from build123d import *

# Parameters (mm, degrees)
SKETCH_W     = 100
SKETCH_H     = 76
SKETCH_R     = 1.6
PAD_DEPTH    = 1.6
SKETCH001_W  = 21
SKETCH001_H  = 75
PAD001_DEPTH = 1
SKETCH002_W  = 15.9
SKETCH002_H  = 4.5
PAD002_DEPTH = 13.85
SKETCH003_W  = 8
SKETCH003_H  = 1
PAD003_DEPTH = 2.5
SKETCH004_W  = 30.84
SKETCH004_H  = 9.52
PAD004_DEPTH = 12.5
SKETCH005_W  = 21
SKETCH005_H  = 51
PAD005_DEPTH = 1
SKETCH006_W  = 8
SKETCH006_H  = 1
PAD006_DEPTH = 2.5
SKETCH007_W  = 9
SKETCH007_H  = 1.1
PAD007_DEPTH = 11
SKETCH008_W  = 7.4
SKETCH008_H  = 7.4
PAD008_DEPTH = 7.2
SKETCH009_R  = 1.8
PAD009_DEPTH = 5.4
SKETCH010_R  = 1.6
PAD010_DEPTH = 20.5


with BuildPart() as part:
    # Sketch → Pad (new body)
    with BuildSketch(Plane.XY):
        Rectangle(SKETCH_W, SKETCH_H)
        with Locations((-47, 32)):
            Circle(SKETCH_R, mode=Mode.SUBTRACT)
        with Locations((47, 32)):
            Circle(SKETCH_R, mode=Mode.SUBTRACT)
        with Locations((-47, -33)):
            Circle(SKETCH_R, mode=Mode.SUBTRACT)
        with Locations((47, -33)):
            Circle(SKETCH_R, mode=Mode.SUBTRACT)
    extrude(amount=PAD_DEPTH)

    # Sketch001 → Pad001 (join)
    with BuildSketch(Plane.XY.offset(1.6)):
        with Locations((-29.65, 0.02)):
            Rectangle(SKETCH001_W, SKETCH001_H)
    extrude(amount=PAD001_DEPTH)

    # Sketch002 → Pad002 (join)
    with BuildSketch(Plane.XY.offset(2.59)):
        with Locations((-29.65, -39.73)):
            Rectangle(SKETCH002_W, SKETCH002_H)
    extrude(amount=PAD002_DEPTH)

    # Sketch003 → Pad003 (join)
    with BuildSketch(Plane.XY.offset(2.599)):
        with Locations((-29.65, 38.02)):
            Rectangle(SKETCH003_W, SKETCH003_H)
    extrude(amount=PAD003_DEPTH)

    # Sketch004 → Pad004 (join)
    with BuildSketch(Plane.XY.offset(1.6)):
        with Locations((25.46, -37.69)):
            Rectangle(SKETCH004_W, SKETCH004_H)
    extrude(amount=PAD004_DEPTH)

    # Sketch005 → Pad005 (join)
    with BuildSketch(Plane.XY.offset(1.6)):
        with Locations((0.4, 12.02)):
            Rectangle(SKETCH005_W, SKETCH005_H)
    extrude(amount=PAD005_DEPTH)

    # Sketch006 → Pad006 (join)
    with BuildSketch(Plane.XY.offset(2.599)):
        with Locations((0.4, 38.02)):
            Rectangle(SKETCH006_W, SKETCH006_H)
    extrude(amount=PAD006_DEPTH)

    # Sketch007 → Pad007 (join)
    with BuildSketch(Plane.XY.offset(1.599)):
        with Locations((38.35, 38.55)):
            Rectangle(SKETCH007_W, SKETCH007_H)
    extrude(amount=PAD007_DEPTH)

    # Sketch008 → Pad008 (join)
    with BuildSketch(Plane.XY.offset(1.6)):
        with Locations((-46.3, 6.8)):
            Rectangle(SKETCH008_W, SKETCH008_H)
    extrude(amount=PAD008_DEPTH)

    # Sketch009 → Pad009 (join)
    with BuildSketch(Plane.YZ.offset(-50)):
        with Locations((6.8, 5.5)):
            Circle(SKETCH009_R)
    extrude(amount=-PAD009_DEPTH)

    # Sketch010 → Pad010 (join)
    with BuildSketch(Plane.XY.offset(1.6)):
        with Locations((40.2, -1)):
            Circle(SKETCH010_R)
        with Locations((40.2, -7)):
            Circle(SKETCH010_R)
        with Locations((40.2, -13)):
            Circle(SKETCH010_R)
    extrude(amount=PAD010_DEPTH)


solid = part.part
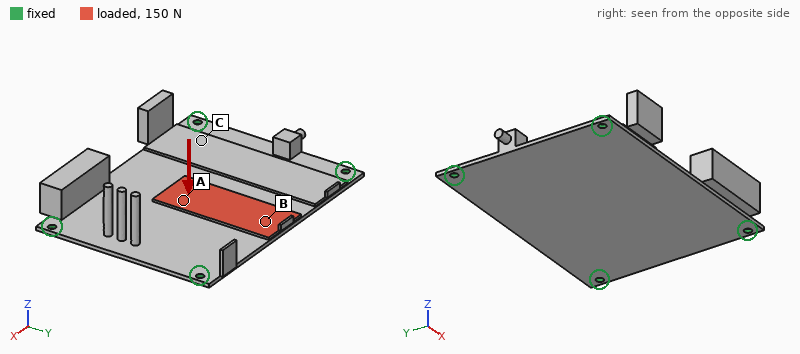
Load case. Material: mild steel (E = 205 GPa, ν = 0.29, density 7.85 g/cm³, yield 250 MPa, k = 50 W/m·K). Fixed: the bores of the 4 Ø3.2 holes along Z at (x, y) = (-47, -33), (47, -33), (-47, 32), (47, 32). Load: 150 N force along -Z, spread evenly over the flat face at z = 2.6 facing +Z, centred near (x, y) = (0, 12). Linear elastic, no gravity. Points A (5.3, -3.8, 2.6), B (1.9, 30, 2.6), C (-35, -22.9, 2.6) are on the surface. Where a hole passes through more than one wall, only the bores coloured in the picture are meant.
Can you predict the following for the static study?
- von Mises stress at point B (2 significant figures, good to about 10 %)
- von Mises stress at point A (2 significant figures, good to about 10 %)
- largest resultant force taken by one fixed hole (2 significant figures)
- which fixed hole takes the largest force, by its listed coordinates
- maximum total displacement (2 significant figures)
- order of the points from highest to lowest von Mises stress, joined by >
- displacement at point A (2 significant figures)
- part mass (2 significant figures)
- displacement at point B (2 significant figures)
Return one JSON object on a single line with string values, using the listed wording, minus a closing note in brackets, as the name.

{"von Mises stress at point B": "29 MPa", "von Mises stress at point A": "20 MPa", "largest resultant force taken by one fixed hole": "120 N", "which fixed hole takes the largest force, by its listed coordinates": "(-47, 32)", "maximum total displacement": "0.13 mm", "order of the points from highest to lowest von Mises stress, joined by >": "B > A > C", "displacement at point A": "0.11 mm", "part mass": "160 g", "displacement at point B": "0.12 mm"}
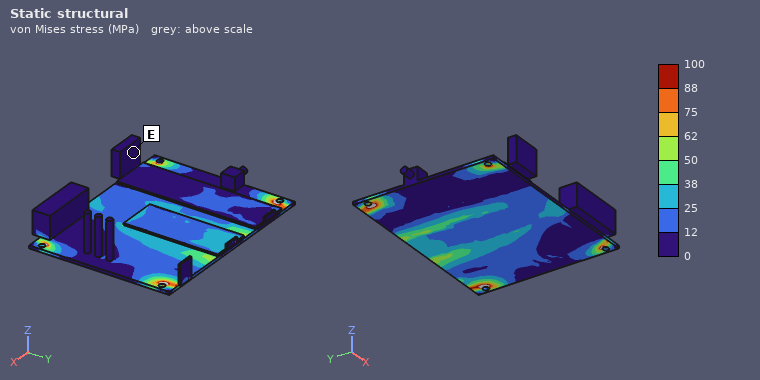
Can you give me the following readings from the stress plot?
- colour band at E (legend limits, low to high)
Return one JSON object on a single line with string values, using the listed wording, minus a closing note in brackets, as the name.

{"colour band at E": "0 to 12 MPa"}
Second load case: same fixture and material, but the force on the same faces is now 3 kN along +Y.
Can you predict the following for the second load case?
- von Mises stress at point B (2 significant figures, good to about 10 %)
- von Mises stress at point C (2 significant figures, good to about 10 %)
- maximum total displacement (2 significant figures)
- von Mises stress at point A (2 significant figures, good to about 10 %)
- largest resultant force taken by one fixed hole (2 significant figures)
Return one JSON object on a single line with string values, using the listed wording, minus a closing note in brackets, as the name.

{"von Mises stress at point B": "30 MPa", "von Mises stress at point C": "33 MPa", "maximum total displacement": "0.13 mm", "von Mises stress at point A": "23 MPa", "largest resultant force taken by one fixed hole": "1.0 kN"}
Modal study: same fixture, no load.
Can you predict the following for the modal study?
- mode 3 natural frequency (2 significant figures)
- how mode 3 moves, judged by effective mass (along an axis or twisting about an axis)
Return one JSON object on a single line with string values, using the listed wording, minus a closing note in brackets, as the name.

{"mode 3 natural frequency": "690 Hz", "how mode 3 moves, judged by effective mass": "along Z"}
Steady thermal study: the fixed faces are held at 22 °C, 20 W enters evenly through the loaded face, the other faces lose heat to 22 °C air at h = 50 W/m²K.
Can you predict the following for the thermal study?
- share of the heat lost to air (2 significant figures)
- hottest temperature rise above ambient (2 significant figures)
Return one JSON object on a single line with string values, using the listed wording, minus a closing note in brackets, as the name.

{"share of the heat lost to air": "75 %", "hottest temperature rise above ambient": "49 K"}
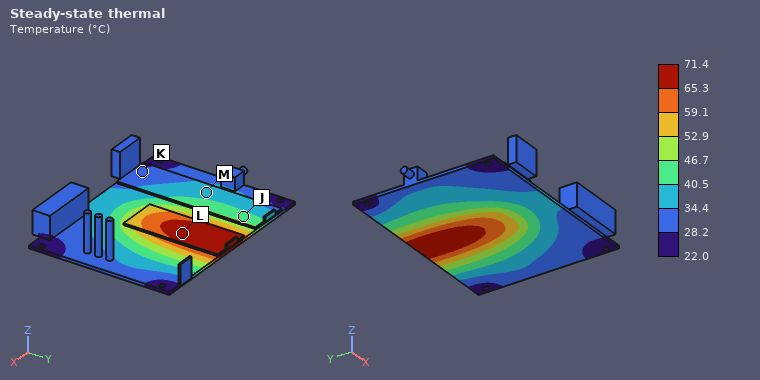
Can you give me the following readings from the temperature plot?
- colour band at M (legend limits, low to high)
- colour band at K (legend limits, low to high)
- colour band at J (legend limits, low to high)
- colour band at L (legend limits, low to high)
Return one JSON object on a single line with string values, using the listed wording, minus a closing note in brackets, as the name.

{"colour band at M": "34.4 to 40.5 °C", "colour band at K": "28.2 to 34.4 °C", "colour band at J": "40.5 to 46.7 °C", "colour band at L": "65.3 to 71.4 °C"}
